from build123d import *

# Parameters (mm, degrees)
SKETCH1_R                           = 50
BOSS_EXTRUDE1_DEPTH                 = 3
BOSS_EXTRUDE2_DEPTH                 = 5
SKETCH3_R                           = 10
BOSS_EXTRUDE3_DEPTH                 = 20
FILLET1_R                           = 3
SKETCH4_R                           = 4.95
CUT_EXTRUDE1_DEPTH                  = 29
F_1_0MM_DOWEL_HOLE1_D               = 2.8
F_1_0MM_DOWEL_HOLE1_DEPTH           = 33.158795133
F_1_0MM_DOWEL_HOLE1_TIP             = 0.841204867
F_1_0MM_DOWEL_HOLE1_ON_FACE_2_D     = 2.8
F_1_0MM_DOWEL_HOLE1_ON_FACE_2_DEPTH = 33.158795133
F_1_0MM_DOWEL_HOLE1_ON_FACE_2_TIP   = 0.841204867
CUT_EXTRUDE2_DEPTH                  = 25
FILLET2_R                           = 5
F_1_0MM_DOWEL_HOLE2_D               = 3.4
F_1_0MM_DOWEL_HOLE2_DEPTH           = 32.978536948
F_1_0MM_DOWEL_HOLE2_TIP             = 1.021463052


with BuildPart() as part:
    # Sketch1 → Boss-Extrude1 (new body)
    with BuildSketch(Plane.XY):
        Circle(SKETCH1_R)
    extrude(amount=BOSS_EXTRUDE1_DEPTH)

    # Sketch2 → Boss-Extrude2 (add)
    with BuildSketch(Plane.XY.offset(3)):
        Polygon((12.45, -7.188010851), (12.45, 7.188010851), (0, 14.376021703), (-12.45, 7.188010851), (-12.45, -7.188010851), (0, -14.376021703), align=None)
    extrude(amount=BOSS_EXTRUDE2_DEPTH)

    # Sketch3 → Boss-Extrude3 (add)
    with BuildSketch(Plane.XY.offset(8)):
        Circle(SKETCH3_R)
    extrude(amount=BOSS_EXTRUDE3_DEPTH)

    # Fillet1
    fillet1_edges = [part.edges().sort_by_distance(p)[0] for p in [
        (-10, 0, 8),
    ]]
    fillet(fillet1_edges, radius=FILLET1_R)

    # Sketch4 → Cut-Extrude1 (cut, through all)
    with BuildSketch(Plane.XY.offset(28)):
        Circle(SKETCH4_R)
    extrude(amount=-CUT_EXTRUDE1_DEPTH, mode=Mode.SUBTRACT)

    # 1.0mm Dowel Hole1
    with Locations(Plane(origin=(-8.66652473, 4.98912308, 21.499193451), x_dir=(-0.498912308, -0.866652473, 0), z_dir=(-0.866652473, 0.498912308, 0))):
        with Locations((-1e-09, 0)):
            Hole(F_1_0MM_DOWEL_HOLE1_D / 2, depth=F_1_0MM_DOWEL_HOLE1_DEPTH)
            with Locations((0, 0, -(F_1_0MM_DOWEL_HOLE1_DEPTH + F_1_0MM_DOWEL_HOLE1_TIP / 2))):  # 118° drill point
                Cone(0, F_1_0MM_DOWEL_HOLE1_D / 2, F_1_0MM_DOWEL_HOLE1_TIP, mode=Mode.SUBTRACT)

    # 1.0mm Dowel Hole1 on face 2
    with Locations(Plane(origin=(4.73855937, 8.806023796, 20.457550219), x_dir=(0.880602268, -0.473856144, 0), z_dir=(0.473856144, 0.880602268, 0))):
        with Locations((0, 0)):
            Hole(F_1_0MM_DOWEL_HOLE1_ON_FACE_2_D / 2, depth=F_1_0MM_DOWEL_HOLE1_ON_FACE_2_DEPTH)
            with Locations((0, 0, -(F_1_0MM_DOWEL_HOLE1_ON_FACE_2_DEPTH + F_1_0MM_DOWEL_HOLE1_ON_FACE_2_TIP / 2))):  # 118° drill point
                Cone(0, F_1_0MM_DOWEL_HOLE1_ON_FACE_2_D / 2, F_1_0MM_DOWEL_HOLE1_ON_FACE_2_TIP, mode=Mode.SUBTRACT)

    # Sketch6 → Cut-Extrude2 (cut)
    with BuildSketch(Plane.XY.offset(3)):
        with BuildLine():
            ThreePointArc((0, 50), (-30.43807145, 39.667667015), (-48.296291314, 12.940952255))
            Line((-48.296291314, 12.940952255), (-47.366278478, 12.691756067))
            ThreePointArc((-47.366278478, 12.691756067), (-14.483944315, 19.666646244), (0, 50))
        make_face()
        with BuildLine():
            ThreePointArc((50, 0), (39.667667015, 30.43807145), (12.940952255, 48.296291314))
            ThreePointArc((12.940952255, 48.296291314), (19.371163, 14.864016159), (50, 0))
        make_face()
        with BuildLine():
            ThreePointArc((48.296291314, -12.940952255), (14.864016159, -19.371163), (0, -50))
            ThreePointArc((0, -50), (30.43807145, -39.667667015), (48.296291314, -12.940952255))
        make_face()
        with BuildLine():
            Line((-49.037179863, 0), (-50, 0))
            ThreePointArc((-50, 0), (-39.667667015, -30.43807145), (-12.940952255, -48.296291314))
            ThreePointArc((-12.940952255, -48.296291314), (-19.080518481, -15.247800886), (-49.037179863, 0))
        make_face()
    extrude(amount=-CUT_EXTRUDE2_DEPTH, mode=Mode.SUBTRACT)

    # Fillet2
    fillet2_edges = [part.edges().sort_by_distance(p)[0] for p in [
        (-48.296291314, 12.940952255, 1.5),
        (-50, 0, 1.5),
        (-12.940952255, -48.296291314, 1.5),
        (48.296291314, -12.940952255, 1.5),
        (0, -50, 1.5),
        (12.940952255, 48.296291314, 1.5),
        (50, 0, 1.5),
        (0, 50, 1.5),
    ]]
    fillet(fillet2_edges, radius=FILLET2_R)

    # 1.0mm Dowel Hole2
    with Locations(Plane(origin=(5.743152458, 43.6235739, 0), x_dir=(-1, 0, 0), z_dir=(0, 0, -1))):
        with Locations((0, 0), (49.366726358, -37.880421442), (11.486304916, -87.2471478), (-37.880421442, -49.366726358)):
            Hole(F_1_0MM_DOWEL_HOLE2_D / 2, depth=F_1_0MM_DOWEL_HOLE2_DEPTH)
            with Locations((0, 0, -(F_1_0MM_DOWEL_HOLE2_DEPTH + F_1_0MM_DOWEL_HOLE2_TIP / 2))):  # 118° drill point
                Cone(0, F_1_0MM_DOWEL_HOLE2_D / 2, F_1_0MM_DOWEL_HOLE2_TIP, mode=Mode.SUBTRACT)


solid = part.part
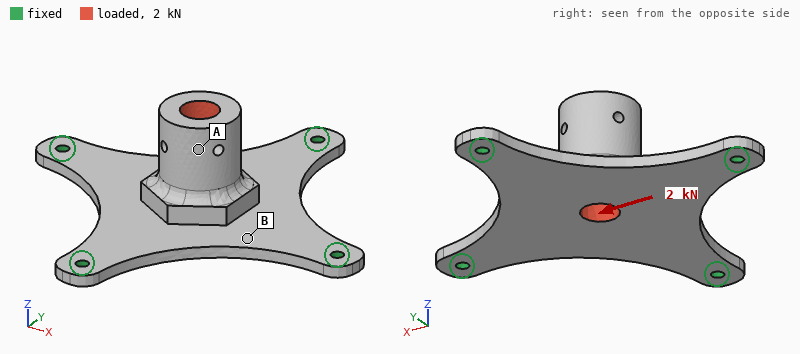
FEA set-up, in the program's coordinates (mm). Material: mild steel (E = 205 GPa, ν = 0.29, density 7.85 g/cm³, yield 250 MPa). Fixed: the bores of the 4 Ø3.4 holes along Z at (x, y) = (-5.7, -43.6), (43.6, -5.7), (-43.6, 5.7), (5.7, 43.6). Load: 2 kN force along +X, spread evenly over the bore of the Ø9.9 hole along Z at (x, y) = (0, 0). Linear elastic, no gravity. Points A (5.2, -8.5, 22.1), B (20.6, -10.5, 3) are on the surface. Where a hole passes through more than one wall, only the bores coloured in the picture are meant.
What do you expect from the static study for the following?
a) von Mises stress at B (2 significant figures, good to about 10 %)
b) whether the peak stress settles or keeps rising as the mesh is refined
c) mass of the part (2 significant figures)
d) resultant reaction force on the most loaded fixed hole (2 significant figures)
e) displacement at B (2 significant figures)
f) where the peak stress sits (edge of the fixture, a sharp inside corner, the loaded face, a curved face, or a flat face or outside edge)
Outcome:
100 MPa
keeps rising
140 g
940 N
0.045 mm
edge of the fixture
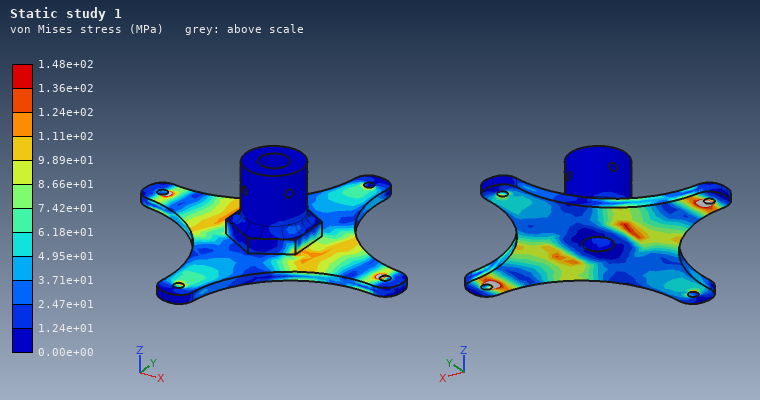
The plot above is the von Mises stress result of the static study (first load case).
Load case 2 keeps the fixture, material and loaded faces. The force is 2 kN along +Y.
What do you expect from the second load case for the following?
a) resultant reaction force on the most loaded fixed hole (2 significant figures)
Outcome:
940 N
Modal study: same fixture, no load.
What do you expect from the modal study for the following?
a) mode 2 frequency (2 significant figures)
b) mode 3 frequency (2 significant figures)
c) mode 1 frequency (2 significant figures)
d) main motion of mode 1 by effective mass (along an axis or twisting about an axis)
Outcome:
3000 Hz
3000 Hz
1800 Hz
along Z
